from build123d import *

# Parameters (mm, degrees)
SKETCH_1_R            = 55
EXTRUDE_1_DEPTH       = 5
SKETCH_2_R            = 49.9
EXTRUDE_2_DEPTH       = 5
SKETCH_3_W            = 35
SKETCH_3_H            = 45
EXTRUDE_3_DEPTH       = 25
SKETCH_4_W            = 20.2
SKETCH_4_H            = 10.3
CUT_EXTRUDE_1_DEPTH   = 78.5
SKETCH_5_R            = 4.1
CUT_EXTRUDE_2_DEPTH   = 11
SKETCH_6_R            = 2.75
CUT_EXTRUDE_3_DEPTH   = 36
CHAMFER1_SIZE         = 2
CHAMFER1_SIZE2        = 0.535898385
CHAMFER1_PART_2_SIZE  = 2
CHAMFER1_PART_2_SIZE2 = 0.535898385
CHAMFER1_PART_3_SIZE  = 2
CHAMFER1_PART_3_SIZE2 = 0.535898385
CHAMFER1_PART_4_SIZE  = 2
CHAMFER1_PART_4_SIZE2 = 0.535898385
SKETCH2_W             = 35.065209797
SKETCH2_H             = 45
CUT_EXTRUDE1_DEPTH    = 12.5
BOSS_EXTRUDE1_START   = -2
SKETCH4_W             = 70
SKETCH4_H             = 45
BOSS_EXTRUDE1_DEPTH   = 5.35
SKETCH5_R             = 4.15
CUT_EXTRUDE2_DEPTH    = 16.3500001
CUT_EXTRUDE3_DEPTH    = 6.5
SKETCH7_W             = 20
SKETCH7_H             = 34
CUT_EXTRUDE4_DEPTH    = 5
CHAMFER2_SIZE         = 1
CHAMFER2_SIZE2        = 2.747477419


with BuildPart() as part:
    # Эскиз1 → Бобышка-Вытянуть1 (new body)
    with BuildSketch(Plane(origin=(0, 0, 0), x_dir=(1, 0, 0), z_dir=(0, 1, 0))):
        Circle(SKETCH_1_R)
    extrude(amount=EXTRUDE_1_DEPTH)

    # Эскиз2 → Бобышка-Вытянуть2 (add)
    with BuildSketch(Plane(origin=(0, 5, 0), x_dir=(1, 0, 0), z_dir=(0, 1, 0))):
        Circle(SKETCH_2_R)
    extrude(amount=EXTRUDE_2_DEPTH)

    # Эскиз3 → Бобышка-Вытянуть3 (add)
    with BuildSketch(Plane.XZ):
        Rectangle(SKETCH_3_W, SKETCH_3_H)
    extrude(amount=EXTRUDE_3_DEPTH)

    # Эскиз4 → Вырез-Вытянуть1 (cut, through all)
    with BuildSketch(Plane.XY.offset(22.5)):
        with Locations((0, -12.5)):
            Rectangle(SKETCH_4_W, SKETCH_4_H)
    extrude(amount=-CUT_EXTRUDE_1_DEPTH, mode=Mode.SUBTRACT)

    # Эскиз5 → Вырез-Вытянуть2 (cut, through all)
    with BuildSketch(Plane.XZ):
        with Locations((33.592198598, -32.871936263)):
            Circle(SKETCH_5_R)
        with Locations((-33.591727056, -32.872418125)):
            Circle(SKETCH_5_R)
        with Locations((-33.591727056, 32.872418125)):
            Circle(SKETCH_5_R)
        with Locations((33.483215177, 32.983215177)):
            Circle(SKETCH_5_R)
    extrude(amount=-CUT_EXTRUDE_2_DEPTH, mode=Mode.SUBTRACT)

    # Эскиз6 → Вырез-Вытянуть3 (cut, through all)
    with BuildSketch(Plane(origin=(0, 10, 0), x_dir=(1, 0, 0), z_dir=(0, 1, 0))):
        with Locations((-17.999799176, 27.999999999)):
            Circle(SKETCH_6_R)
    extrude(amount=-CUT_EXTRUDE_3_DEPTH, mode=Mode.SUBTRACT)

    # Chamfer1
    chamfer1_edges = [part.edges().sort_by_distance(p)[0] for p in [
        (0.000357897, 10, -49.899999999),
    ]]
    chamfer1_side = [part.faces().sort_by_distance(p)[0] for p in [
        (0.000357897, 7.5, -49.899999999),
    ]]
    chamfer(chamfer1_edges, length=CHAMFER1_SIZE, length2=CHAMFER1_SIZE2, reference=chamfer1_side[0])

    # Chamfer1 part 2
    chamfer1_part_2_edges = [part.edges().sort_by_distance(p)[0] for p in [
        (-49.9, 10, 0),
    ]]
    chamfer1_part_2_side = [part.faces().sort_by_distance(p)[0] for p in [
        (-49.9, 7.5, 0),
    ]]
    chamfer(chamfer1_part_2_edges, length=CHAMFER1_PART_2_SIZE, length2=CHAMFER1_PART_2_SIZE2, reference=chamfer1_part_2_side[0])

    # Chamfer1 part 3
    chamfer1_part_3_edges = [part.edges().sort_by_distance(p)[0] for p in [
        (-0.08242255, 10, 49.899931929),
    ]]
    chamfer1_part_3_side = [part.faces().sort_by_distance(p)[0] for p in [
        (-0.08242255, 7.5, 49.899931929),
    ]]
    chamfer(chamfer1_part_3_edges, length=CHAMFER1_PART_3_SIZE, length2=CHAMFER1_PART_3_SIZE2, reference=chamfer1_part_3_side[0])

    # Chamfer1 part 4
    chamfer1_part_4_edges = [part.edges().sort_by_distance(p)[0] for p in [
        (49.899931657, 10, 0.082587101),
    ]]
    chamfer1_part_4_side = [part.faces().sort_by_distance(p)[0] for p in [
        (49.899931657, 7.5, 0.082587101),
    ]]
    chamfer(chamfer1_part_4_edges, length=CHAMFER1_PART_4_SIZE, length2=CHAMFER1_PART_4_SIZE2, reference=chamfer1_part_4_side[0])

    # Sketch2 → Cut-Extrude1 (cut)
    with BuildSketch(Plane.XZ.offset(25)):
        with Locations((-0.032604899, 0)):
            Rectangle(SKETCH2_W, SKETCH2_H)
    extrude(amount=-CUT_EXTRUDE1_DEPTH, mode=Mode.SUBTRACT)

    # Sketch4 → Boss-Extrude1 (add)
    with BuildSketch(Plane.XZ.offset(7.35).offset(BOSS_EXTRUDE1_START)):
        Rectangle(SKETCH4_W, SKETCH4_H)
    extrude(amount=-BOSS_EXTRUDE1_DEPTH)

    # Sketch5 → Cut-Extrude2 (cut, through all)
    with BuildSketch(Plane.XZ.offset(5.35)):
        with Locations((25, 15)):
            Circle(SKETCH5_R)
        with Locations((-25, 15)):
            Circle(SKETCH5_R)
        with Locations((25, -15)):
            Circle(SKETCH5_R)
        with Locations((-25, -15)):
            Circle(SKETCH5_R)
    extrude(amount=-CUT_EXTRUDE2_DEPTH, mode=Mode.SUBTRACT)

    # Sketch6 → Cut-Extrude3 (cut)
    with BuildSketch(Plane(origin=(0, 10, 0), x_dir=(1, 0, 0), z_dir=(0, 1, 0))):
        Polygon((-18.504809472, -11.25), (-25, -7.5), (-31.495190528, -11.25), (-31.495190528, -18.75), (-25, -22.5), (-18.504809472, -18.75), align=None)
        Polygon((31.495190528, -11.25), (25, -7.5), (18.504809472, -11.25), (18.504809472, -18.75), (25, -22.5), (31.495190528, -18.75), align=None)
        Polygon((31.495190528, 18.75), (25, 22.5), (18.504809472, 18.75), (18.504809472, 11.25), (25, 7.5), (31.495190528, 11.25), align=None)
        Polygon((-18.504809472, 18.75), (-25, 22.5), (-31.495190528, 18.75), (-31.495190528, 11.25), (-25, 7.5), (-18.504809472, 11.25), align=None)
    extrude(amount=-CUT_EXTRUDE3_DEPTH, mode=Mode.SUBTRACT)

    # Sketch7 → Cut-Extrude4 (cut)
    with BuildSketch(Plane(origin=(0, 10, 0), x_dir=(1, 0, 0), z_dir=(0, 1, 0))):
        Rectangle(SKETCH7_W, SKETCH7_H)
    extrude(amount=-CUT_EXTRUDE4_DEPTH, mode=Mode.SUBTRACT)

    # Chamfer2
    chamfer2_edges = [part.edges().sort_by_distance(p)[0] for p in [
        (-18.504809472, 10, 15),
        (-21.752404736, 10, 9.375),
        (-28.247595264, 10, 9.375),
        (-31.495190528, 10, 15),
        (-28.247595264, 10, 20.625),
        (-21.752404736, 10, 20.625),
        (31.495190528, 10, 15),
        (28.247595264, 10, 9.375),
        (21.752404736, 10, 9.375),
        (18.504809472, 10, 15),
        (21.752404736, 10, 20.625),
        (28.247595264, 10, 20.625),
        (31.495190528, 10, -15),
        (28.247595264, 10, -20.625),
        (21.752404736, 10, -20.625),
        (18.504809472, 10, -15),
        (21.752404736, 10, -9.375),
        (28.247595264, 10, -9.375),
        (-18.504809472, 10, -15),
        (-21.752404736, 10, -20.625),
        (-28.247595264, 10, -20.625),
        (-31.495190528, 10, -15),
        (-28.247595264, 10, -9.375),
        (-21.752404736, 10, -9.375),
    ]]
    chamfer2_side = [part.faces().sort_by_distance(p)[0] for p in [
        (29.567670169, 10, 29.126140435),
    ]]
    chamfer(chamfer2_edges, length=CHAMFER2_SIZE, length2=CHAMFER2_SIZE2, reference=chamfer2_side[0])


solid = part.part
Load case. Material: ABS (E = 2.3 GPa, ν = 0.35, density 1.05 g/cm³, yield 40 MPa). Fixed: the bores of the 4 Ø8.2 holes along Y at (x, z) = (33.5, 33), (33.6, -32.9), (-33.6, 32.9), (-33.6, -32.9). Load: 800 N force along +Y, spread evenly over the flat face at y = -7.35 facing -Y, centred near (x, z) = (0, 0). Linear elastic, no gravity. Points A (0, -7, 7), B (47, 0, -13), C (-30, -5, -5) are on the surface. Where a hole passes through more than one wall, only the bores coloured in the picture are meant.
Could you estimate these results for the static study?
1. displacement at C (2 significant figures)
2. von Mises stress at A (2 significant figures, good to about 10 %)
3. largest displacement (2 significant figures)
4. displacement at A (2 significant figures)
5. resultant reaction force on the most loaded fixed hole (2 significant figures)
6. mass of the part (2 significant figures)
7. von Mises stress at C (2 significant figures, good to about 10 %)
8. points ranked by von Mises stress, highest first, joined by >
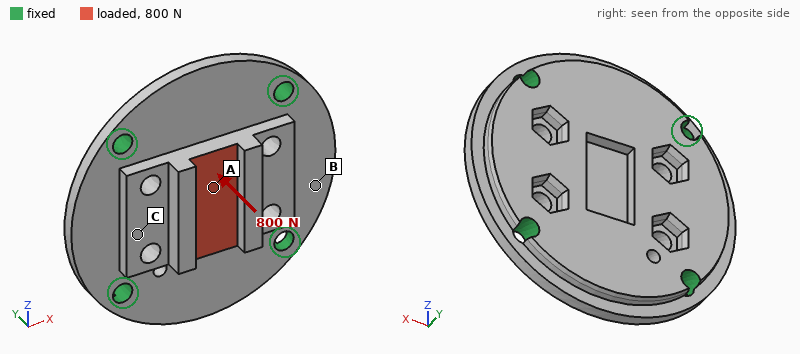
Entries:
0.042 mm
2.5 MPa
0.10 mm
0.100 mm
240 N
100 g
1.3 MPa
A > C > B
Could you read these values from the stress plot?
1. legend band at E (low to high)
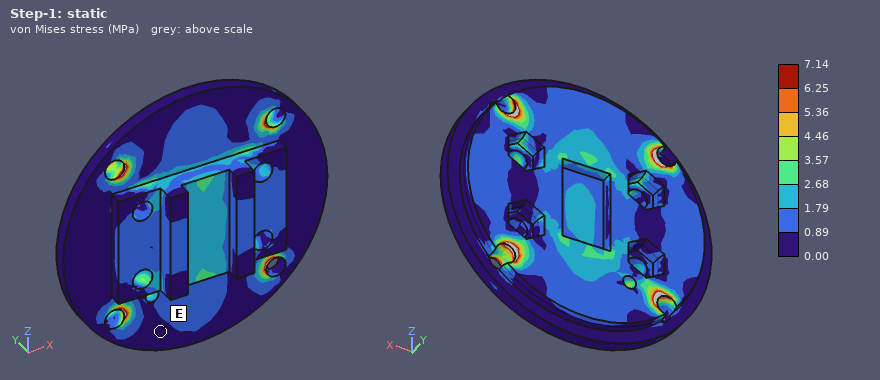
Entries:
0.00 to 0.89 MPa
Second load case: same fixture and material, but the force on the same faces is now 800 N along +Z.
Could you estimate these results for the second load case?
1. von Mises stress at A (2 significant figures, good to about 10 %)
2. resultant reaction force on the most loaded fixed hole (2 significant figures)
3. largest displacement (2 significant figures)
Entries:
1.5 MPa
230 N
45 µm
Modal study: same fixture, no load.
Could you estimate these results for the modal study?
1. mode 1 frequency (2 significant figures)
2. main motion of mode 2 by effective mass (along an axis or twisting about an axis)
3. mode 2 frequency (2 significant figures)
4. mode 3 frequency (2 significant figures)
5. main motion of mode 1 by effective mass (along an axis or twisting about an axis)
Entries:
2400 Hz
twisting about X
2800 Hz
2900 Hz
along Y
